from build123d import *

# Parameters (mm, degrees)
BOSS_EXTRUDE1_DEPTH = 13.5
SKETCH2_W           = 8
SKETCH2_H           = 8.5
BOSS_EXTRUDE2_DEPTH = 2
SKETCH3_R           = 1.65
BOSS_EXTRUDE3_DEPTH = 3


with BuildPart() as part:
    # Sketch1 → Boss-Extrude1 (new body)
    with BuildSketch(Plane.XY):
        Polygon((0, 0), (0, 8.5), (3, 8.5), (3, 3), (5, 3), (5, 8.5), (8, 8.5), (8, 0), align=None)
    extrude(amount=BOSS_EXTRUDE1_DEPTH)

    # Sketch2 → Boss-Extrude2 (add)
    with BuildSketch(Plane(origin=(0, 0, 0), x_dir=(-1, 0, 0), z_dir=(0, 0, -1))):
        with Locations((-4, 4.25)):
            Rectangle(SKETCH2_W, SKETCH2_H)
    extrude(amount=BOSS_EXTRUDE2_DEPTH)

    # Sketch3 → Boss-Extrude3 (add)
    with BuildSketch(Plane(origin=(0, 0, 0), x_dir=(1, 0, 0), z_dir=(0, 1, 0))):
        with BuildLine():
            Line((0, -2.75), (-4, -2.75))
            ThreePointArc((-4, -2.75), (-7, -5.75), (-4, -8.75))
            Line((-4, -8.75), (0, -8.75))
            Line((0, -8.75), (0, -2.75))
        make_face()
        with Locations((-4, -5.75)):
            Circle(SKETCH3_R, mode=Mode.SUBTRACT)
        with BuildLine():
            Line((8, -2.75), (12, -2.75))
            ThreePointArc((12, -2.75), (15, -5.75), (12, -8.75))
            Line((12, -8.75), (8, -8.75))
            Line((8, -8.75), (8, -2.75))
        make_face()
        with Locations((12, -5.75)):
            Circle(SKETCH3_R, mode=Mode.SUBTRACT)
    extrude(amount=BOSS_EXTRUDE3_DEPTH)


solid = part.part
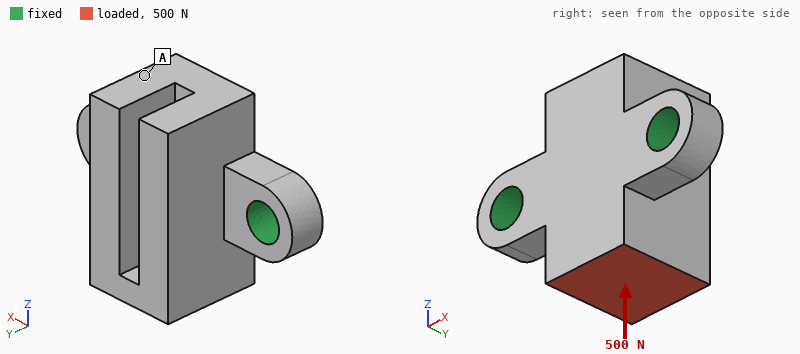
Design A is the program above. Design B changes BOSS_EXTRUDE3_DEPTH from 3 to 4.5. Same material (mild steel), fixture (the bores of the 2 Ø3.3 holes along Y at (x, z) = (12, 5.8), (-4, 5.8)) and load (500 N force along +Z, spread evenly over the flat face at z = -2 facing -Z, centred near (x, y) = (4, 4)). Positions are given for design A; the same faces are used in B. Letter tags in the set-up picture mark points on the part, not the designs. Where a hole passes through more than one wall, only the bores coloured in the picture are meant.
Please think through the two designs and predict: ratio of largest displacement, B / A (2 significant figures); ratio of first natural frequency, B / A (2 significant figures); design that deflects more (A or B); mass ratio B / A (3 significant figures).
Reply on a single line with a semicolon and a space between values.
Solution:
0.37; 1.6; A; 1.08
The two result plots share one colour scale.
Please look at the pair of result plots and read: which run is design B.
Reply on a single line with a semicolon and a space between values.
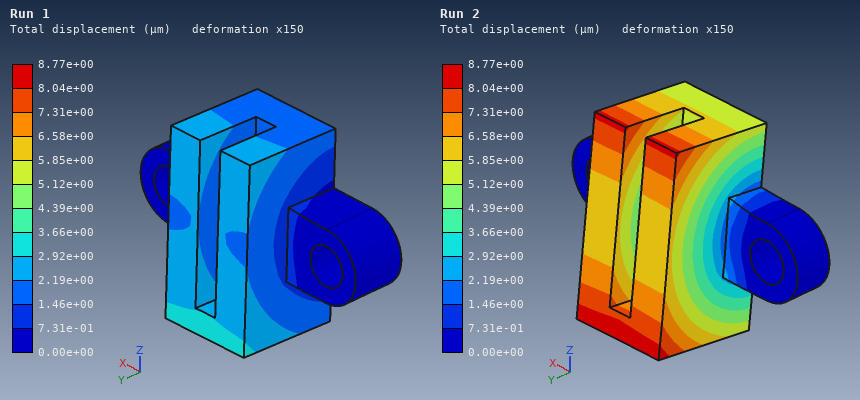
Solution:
Run 1
